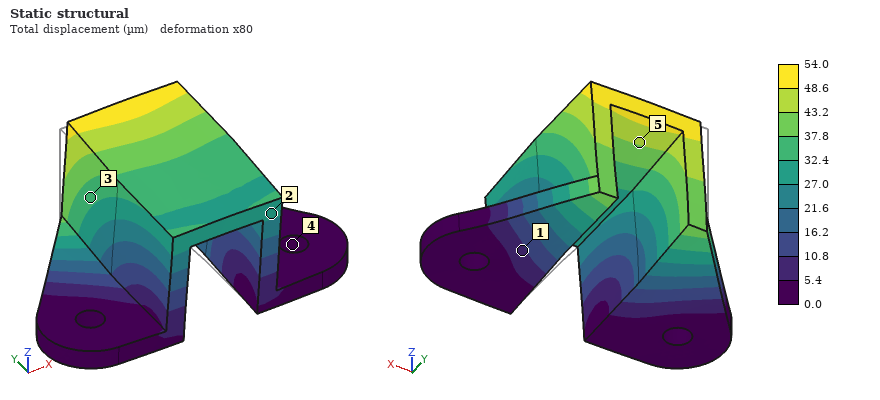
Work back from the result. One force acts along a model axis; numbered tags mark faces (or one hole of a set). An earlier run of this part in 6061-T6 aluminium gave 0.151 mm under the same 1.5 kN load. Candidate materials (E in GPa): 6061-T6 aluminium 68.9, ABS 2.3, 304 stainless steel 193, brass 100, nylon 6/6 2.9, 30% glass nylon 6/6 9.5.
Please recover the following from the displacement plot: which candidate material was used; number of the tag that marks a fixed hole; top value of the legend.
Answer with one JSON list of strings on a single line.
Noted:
["304 stainless steel", "4", "54.0 µm"]
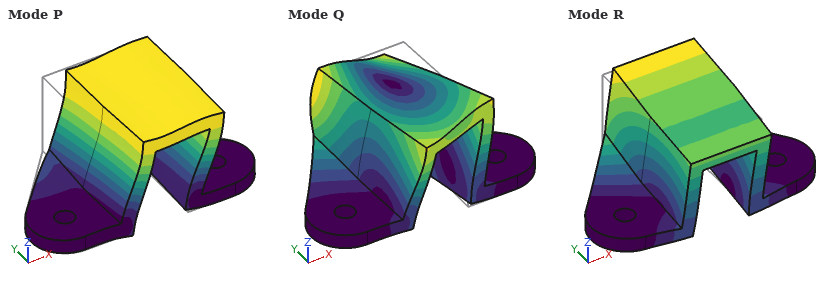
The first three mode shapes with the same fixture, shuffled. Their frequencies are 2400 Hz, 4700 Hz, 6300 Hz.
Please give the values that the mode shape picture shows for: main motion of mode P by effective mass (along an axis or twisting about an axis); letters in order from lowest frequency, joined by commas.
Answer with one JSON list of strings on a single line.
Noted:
["along X", "R, P, Q"]
